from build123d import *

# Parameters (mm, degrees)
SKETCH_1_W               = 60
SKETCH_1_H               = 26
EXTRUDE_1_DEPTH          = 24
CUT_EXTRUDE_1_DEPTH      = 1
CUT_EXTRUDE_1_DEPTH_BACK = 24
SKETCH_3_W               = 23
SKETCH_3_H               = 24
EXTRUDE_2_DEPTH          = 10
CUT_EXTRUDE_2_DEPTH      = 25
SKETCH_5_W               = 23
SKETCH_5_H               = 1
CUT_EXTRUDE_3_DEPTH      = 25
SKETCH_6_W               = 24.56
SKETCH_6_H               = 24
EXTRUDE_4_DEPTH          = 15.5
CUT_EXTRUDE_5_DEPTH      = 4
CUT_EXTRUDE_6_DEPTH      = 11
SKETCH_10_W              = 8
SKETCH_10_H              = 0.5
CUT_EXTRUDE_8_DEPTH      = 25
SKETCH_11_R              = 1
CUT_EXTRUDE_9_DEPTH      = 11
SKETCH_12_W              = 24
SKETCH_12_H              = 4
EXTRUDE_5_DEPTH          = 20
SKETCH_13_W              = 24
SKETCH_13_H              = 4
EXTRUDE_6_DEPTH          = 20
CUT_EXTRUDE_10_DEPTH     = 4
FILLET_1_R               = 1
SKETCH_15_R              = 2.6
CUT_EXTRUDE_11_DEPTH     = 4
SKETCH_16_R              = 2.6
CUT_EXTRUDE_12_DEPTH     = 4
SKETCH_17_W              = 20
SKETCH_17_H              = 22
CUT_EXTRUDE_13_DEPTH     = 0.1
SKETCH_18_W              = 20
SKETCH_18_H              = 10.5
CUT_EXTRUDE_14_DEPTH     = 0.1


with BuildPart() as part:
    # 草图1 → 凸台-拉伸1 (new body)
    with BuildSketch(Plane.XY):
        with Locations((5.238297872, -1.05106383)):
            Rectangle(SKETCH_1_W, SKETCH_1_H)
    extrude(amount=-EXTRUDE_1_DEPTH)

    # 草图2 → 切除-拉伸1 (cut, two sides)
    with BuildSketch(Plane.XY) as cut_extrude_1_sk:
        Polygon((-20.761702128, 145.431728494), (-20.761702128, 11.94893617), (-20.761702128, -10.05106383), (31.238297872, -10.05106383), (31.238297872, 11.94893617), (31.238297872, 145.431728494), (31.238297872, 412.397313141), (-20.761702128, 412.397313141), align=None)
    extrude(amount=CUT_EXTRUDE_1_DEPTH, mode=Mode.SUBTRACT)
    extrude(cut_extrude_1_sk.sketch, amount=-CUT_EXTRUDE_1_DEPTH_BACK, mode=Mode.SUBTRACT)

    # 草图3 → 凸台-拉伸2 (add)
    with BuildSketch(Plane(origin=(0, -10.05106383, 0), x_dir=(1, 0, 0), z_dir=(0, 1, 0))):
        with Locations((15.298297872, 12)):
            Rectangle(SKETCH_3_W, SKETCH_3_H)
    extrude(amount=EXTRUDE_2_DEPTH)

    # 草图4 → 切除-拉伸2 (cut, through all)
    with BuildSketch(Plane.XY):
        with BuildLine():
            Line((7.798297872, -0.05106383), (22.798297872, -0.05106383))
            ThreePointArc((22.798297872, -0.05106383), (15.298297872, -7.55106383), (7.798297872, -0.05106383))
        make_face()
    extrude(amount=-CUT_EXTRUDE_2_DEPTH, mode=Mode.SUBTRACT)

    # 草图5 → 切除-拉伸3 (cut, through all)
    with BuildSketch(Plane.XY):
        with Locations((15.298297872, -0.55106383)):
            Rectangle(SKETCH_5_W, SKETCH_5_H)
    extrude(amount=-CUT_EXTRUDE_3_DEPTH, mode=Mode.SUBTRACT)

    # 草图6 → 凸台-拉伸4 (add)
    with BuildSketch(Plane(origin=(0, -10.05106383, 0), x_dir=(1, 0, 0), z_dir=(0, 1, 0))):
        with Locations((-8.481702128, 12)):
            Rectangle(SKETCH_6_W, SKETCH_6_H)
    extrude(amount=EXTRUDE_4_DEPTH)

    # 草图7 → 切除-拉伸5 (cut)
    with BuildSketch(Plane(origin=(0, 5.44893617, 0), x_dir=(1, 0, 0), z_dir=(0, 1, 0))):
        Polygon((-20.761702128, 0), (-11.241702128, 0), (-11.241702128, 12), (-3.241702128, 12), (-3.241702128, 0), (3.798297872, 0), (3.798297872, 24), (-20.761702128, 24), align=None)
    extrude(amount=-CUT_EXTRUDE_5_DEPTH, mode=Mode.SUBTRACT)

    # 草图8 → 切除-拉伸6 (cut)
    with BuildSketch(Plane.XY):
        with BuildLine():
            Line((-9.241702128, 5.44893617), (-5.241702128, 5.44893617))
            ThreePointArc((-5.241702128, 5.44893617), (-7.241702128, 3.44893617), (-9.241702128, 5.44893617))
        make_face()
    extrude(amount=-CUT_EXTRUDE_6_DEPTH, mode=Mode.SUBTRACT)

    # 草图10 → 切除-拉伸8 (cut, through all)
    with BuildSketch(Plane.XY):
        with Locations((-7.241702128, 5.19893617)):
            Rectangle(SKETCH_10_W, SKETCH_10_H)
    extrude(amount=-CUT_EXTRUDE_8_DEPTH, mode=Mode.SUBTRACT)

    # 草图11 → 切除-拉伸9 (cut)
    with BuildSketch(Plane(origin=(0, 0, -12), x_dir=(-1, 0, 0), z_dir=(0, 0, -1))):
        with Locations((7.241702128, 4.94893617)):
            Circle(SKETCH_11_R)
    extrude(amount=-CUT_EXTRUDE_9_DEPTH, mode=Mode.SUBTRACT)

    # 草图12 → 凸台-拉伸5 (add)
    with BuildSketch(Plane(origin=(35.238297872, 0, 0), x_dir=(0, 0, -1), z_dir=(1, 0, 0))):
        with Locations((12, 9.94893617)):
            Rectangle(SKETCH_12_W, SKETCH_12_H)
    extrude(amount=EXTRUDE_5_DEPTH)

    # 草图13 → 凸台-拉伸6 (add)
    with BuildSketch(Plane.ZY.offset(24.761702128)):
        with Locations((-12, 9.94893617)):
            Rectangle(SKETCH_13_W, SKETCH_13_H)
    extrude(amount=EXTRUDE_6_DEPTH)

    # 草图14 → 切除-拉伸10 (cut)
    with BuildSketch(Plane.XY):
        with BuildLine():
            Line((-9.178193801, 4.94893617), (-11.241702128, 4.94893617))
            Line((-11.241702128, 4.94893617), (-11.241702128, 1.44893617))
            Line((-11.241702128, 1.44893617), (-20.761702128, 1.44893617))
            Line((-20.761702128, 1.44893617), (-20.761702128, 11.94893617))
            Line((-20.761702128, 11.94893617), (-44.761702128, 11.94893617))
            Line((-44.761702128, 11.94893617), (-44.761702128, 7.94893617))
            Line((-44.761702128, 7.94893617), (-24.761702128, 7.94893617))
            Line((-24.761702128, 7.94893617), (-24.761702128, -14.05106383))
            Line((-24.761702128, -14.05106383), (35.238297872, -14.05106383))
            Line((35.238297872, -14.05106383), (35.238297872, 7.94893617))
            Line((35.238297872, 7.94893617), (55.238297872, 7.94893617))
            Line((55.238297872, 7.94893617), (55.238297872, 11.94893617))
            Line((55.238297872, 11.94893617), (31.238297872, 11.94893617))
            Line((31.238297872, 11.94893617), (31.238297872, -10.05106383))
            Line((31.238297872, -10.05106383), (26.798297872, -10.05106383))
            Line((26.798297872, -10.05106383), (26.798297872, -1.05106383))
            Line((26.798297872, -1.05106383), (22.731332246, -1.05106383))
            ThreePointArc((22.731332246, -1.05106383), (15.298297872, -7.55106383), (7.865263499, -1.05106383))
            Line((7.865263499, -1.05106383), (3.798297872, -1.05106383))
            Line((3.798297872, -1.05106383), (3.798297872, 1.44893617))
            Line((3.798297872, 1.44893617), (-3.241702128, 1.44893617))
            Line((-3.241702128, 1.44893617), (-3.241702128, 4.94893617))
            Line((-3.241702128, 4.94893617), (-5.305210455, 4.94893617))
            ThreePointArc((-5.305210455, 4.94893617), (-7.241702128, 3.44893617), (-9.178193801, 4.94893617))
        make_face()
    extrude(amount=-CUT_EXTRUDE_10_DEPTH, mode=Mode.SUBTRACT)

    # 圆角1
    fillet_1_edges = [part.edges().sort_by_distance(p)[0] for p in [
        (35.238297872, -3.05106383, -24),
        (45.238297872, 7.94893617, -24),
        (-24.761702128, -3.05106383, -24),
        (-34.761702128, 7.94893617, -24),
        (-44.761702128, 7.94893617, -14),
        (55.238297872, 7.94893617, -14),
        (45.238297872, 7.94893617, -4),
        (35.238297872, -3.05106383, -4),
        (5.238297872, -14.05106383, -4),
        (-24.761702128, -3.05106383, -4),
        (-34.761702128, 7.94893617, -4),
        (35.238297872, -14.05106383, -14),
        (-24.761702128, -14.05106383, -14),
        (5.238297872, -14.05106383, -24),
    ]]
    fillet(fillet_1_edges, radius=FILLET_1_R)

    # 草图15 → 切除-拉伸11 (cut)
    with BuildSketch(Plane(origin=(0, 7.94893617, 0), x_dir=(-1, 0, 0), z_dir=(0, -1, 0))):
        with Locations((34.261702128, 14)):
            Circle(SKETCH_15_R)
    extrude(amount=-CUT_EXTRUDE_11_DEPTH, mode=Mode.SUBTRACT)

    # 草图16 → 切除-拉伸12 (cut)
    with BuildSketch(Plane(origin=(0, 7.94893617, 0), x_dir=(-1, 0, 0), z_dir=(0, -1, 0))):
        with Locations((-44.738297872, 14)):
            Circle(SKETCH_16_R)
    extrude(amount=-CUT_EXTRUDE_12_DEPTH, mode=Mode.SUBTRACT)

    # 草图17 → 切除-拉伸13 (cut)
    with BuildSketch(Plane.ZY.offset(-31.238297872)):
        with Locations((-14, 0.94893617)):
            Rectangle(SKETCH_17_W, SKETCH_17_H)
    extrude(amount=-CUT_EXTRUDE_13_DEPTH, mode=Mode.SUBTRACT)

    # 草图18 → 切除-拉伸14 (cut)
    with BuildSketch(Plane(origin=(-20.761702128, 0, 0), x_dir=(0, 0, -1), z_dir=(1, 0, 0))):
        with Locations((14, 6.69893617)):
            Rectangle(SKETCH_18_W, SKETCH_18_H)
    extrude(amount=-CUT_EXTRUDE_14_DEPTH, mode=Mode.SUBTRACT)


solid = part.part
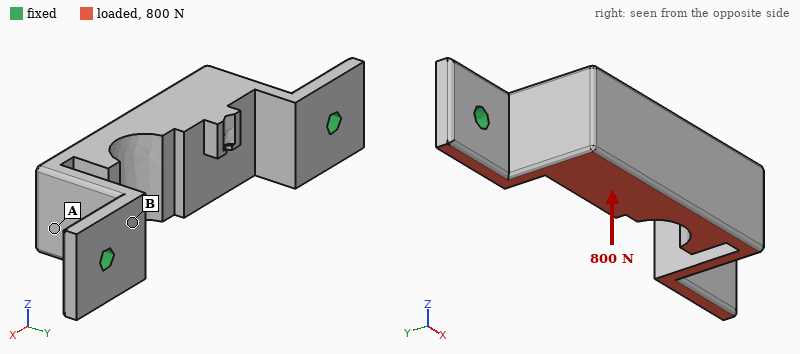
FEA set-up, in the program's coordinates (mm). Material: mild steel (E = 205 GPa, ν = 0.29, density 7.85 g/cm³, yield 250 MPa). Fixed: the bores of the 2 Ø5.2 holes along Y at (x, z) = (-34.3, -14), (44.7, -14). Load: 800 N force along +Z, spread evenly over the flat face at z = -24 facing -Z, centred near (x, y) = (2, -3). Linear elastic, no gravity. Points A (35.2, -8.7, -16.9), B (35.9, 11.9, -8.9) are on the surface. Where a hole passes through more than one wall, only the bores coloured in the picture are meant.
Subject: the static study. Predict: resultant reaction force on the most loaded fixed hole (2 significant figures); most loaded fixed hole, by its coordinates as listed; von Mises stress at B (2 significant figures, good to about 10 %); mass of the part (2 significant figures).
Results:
450 N
(-34.3, -14)
41 MPa
150 g
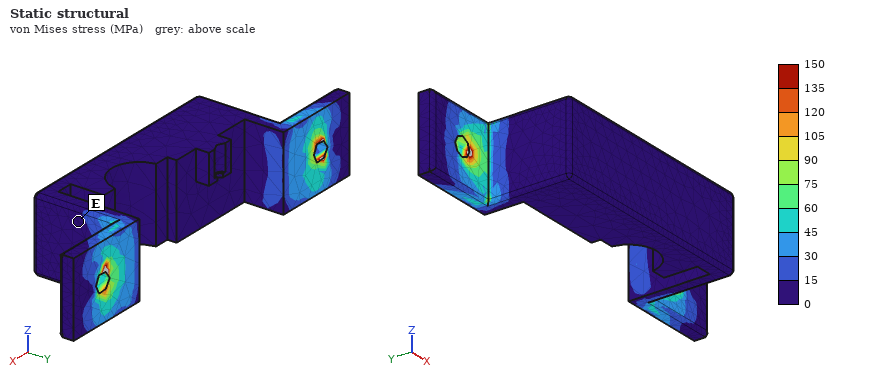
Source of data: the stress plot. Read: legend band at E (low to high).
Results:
0 to 15 MPa
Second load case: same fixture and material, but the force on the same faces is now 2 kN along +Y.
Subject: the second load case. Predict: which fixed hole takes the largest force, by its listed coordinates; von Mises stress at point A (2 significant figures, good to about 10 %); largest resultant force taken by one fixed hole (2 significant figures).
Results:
(-34.3, -14)
44 MPa
1.2 kN
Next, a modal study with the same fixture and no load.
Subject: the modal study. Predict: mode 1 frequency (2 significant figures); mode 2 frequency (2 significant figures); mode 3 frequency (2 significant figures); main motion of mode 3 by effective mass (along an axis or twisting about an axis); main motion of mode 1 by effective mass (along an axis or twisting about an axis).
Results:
2100 Hz
3900 Hz
5400 Hz
twisting about Y
along Z
